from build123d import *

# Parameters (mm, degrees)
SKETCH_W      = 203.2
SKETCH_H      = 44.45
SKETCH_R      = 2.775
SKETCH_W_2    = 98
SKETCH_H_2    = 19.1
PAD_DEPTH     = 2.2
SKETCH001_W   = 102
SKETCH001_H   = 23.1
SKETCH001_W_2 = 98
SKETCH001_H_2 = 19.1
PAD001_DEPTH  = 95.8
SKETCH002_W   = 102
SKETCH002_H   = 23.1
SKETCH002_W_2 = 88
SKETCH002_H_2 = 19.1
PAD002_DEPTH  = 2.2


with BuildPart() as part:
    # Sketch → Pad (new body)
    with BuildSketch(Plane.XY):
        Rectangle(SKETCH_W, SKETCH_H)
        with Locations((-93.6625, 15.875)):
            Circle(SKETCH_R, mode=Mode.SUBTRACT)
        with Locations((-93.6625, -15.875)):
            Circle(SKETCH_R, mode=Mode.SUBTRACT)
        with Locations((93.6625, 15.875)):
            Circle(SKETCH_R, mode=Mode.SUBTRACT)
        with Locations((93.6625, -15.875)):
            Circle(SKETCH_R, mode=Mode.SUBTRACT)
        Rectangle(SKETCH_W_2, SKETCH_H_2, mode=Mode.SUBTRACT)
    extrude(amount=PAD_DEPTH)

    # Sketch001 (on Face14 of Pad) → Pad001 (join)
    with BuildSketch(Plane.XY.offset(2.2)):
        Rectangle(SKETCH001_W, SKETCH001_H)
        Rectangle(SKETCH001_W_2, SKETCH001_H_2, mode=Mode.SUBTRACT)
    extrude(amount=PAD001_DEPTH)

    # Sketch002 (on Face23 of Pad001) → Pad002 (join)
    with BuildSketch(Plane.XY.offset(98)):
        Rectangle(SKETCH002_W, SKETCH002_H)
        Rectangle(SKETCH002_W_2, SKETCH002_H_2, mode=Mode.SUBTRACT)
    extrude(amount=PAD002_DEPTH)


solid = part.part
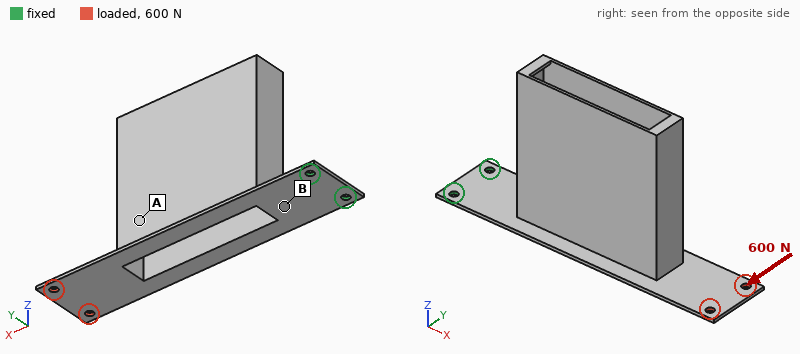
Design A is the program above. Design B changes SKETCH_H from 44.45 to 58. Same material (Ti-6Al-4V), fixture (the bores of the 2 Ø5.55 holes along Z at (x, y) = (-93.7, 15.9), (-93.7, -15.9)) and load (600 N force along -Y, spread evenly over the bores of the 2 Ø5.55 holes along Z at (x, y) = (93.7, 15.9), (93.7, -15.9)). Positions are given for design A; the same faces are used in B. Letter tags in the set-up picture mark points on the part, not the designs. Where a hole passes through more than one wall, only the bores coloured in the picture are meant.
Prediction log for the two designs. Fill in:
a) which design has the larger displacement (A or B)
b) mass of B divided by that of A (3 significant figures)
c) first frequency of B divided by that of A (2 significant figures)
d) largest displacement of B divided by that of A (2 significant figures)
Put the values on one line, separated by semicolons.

A; 1.10; 1.1; 0.48
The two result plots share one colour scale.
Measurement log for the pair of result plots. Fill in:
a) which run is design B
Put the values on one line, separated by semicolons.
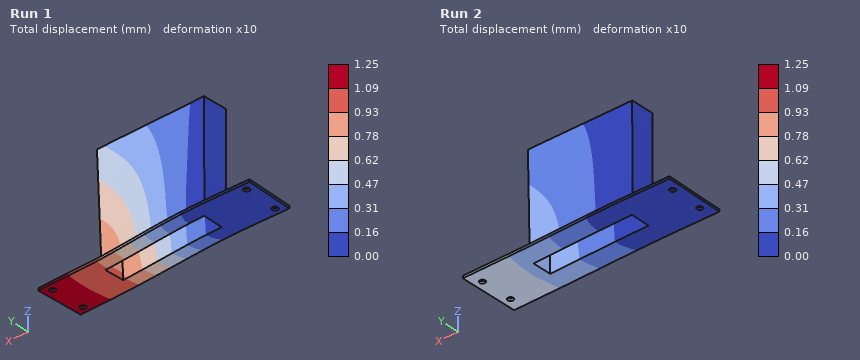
Run 2
